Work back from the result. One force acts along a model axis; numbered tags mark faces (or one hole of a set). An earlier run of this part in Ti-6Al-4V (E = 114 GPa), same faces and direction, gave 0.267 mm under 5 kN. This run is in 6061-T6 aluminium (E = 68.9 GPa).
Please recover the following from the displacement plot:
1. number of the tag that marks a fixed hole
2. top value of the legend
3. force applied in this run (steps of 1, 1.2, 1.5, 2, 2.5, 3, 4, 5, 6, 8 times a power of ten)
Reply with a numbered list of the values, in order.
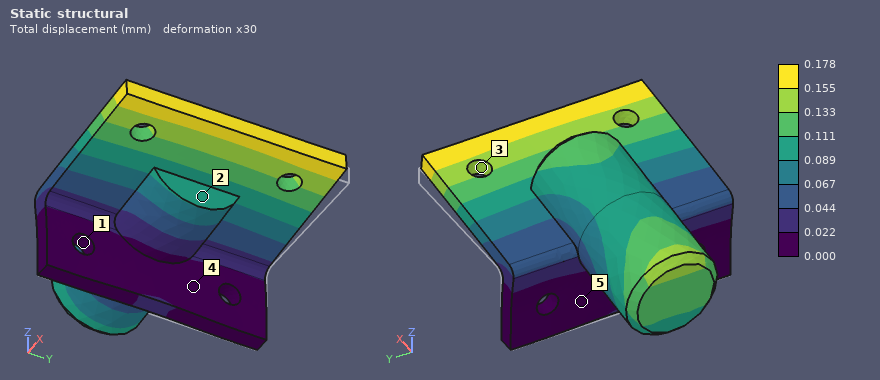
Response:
1. 1
2. 0.178 mm
3. 2 kN
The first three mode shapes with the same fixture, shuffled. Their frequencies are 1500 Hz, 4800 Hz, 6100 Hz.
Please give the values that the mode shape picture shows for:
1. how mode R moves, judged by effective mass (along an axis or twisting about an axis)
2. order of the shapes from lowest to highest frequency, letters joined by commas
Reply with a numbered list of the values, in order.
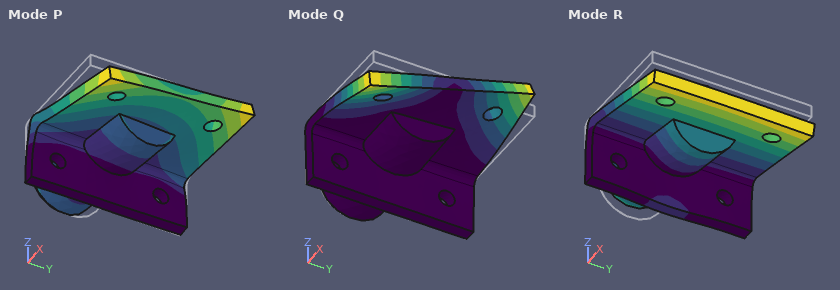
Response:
1. along X
2. R, P, Q
